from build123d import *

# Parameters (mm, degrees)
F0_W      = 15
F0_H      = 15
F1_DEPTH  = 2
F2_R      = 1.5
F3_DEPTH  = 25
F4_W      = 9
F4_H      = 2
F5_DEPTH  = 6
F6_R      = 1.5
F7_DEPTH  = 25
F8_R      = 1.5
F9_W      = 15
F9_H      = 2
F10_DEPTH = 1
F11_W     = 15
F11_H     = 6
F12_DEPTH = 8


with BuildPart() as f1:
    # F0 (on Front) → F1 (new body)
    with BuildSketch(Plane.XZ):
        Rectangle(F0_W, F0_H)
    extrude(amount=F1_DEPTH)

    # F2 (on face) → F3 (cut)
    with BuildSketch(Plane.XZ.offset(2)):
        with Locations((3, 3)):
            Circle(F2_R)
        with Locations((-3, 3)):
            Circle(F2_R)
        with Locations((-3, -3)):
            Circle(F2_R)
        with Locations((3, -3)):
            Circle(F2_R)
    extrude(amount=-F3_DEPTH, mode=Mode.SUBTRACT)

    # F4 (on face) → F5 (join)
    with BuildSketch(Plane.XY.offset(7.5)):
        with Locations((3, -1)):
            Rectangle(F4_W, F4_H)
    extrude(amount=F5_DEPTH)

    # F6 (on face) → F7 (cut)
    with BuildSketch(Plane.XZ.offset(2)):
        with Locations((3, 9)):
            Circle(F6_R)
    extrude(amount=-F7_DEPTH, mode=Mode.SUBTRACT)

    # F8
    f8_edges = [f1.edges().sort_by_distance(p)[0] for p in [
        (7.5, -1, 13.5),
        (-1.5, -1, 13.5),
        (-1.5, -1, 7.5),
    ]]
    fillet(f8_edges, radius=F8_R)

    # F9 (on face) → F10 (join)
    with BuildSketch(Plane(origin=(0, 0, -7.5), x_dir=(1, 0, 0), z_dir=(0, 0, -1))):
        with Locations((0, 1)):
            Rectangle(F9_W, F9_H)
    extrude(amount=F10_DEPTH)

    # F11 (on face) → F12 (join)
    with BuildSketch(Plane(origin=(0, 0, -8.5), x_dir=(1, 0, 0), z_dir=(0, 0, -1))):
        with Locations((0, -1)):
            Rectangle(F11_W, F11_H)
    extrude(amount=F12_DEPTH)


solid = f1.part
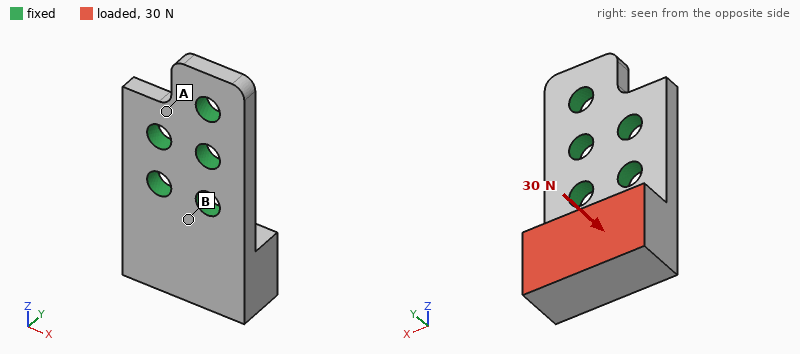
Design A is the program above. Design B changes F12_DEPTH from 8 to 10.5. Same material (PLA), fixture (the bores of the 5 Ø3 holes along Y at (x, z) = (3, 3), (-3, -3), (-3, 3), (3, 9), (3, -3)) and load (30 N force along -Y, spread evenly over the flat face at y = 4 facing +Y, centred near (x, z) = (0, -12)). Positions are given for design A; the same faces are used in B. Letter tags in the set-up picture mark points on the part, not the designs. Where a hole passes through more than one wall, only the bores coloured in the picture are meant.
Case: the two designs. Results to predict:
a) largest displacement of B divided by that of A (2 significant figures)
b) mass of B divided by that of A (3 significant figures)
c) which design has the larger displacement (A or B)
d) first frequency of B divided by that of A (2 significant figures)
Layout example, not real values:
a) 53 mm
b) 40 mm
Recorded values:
a) 1.4
b) 1.18
c) B
d) 0.74
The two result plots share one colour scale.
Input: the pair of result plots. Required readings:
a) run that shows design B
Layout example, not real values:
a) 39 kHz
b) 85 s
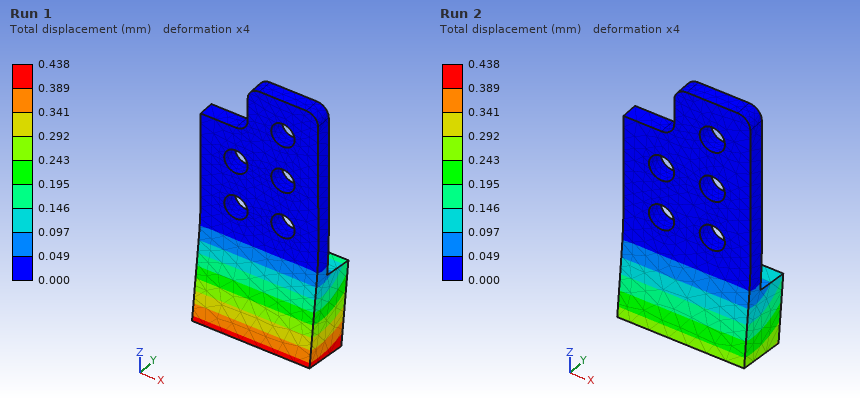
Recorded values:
a) Run 1
